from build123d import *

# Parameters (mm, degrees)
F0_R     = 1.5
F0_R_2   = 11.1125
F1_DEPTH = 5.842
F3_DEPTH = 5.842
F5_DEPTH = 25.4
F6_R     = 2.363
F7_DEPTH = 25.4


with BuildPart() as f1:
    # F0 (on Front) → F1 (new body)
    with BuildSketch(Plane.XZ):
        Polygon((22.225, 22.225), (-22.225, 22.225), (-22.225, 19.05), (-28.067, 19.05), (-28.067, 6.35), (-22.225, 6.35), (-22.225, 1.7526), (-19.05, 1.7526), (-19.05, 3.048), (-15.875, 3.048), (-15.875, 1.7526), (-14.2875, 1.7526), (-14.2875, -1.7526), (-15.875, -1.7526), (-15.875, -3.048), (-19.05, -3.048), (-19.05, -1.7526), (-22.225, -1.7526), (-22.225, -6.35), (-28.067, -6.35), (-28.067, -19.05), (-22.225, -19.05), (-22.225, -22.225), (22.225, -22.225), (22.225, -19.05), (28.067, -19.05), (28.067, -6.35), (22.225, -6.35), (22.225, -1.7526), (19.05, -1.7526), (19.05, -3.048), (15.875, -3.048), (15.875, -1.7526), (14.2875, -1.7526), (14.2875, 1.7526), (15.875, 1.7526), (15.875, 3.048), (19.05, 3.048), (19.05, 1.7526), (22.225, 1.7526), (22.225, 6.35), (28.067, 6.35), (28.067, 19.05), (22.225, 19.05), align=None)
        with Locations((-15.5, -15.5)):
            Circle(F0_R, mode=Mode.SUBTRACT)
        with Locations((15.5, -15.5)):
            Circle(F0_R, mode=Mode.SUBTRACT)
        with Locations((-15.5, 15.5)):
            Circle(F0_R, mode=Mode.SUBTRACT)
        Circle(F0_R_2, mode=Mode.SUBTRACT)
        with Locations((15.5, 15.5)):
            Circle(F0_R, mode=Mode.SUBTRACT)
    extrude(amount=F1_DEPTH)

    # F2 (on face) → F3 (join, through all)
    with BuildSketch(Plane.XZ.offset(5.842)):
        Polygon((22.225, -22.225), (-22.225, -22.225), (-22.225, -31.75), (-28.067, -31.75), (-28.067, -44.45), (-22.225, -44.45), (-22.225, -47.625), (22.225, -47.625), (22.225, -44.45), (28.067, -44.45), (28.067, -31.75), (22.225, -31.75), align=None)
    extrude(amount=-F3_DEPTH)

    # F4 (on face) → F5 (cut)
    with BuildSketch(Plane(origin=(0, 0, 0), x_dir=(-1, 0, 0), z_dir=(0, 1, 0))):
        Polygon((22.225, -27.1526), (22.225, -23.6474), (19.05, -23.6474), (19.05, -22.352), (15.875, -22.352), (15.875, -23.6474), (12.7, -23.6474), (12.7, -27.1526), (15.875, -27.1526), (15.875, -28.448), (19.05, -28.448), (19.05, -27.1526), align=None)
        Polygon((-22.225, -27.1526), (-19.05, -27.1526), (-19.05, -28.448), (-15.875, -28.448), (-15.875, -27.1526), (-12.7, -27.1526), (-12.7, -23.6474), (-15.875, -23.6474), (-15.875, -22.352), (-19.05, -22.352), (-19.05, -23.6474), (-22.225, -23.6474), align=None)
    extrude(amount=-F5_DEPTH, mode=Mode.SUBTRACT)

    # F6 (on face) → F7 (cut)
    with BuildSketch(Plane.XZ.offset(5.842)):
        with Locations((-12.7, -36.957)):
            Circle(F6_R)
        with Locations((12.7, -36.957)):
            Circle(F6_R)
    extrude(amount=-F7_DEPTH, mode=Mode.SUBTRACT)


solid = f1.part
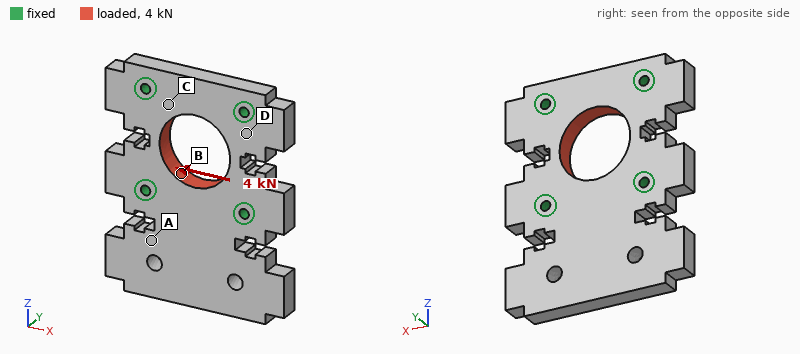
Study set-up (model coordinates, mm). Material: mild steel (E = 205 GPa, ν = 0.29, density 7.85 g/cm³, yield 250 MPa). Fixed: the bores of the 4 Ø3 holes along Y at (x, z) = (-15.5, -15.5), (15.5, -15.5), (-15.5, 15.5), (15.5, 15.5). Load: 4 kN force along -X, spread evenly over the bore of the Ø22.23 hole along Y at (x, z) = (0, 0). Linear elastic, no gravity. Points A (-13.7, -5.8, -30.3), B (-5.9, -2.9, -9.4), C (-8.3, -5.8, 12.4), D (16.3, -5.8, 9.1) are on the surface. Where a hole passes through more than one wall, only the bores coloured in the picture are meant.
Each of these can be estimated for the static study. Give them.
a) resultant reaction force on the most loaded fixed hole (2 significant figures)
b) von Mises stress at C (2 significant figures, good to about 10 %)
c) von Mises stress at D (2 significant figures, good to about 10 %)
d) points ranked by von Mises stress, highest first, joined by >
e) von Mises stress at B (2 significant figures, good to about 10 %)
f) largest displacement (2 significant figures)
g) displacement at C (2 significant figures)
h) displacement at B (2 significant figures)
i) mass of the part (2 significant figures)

1.1 kN
16 MPa
9.6 MPa
B > C > D > A
24 MPa
2.7 µm
0.72 µm
1.1 µm
130 g
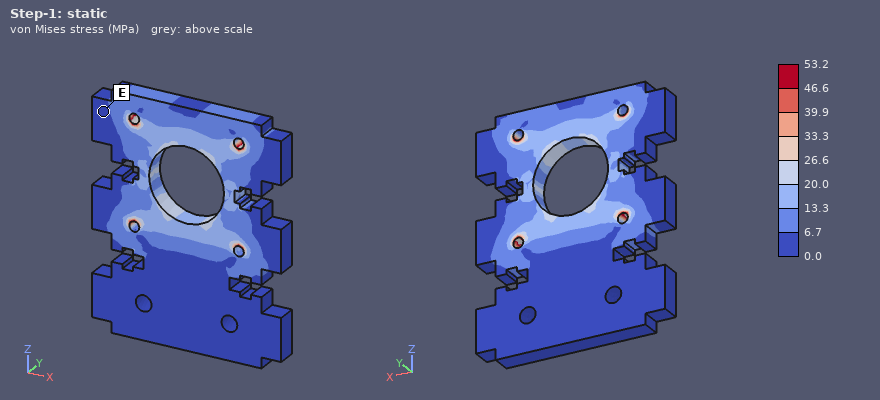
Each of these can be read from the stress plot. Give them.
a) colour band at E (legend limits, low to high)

0.0 to 6.7 MPa
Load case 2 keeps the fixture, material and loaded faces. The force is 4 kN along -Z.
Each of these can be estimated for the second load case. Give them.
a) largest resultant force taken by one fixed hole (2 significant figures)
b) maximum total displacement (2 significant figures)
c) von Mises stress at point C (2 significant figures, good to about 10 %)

1.1 kN
2.5 µm
13 MPa
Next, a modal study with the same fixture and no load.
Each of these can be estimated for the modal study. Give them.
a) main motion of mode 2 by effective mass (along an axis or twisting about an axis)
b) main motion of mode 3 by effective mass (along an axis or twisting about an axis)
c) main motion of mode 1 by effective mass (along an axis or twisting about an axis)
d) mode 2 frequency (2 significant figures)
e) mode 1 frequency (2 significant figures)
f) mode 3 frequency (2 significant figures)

twisting about Z
along X
along Y
4700 Hz
3000 Hz
9800 Hz
